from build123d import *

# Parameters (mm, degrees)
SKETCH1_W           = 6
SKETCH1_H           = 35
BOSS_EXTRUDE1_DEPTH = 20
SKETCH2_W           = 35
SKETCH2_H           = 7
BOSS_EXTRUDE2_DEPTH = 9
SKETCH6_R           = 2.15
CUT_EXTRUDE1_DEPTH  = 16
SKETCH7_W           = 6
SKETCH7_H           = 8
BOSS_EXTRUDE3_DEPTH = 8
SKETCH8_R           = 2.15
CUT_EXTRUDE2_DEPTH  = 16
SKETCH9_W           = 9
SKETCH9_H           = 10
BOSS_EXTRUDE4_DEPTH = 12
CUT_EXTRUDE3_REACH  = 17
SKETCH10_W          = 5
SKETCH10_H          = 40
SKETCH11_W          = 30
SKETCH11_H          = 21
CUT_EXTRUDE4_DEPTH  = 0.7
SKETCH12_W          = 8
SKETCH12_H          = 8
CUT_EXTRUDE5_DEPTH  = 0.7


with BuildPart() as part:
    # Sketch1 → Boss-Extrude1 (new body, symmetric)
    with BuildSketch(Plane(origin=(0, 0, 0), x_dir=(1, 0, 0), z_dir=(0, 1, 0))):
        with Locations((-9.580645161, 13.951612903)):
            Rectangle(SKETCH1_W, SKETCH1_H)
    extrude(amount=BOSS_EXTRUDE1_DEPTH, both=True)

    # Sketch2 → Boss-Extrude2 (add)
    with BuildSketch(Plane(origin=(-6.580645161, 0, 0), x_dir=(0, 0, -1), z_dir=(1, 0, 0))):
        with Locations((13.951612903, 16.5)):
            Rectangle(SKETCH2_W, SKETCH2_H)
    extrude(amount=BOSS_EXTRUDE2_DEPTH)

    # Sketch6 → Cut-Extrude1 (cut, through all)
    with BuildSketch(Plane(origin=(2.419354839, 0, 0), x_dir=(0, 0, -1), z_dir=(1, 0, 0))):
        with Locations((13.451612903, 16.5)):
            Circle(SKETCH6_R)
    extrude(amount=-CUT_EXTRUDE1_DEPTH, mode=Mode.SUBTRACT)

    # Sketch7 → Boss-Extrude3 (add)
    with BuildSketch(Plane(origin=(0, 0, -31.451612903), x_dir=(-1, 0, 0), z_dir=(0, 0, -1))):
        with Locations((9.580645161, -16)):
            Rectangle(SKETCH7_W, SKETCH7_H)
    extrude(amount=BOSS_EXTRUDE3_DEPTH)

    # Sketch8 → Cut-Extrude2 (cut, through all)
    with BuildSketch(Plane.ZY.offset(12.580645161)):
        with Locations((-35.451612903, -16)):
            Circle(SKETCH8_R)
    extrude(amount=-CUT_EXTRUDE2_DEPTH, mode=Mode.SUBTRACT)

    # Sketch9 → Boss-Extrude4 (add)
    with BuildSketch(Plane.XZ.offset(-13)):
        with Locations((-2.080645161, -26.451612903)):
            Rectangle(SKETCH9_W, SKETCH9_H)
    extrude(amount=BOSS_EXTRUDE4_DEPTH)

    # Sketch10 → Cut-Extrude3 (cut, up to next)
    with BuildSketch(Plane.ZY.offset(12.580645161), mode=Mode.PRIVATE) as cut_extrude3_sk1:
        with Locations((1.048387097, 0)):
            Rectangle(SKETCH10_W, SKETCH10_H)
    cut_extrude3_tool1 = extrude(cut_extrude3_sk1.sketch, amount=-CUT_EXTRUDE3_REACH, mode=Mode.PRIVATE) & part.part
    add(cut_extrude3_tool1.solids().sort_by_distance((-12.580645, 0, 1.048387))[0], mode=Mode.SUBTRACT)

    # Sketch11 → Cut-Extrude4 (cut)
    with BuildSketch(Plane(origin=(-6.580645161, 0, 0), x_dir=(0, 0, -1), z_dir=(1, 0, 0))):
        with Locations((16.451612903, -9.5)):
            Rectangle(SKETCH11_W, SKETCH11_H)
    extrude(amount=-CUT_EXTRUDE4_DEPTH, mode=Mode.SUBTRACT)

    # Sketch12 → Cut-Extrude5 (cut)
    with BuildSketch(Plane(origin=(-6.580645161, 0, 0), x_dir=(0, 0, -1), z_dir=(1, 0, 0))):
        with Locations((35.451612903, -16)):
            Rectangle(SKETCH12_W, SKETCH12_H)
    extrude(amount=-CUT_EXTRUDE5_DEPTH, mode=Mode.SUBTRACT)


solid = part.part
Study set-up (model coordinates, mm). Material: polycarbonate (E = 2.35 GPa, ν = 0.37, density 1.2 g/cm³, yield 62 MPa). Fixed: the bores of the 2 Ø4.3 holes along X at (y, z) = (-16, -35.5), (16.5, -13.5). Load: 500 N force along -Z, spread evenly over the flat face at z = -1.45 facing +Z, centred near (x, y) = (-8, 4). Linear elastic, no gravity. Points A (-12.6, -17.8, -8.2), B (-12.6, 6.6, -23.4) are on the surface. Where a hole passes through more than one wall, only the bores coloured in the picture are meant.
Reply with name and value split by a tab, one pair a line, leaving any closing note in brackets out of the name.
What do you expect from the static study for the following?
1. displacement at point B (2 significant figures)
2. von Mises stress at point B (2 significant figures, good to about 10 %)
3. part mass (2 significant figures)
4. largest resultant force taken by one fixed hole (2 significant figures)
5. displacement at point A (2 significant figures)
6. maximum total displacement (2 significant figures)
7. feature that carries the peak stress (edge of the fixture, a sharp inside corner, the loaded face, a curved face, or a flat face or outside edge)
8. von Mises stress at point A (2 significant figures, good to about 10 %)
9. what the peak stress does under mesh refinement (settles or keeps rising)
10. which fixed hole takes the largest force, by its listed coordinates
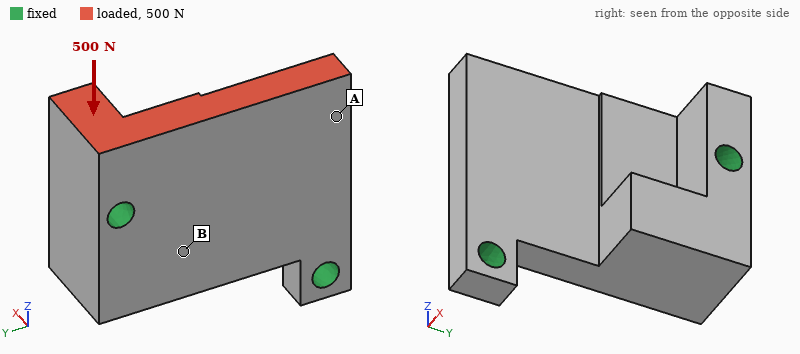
displacement at point B	18 µm
von Mises stress at point B	0.88 MPa
part mass	12 g
largest resultant force taken by one fixed hole	310 N
displacement at point A	37 µm
maximum total displacement	44 µm
feature that carries the peak stress	edge of the fixture
von Mises stress at point A	2.0 MPa
what the peak stress does under mesh refinement	keeps rising
which fixed hole takes the largest force, by its listed coordinates	(16.5, -13.5)
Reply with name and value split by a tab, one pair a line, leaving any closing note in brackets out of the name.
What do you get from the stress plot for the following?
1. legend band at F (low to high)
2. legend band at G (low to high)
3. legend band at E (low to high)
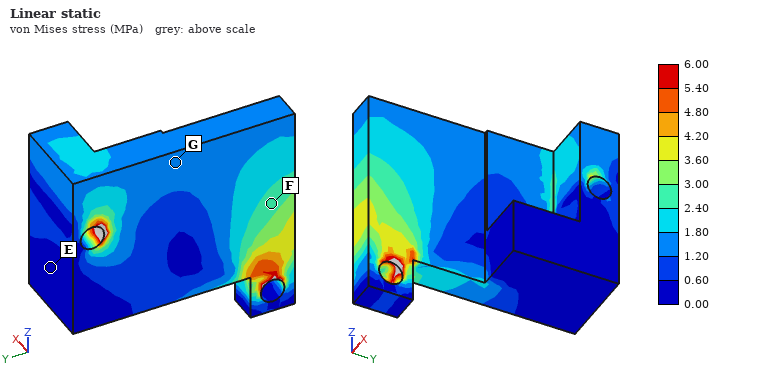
legend band at F	2.40 to 3.00 MPa
legend band at G	1.20 to 1.80 MPa
legend band at E	0.00 to 0.60 MPa
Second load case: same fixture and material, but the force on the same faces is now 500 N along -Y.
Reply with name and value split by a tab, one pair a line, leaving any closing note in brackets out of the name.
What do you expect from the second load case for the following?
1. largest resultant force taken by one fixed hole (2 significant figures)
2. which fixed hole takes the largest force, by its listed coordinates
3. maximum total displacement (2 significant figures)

largest resultant force taken by one fixed hole	490 N
which fixed hole takes the largest force, by its listed coordinates	(16.5, -13.5)
maximum total displacement	92 µm
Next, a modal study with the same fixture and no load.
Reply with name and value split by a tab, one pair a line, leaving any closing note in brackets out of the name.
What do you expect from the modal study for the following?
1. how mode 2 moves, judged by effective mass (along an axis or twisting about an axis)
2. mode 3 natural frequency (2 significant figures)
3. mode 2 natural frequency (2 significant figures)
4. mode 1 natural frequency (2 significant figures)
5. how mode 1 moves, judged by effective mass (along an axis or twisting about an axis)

how mode 2 moves, judged by effective mass	along X
mode 3 natural frequency	5600 Hz
mode 2 natural frequency	4600 Hz
mode 1 natural frequency	2000 Hz
how mode 1 moves, judged by effective mass	along X
